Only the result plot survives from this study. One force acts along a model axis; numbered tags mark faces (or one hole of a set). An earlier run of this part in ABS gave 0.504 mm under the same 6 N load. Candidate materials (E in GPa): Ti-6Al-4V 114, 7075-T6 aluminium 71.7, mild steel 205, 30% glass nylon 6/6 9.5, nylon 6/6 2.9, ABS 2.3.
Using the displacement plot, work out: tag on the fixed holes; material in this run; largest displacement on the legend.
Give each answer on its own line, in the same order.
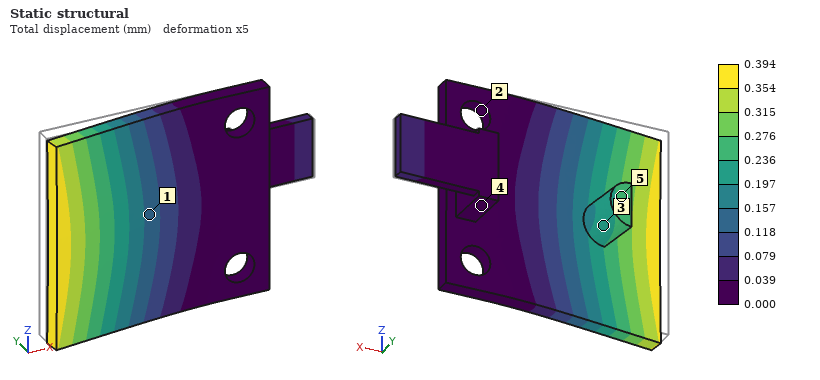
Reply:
2
nylon 6/6
0.394 mm
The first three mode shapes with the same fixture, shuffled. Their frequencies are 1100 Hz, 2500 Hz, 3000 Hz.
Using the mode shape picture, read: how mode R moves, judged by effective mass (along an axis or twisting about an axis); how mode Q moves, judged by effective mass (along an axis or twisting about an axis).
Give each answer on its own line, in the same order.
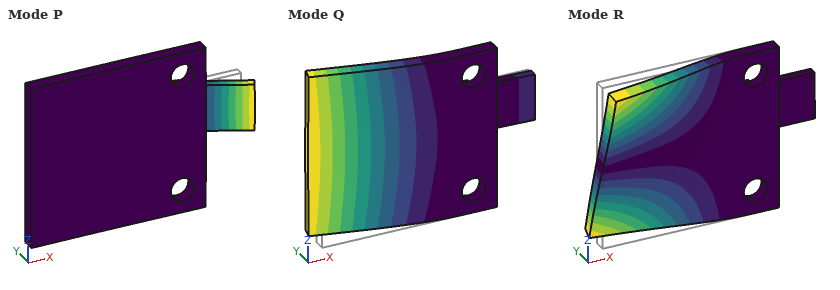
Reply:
twisting about X
along Y
